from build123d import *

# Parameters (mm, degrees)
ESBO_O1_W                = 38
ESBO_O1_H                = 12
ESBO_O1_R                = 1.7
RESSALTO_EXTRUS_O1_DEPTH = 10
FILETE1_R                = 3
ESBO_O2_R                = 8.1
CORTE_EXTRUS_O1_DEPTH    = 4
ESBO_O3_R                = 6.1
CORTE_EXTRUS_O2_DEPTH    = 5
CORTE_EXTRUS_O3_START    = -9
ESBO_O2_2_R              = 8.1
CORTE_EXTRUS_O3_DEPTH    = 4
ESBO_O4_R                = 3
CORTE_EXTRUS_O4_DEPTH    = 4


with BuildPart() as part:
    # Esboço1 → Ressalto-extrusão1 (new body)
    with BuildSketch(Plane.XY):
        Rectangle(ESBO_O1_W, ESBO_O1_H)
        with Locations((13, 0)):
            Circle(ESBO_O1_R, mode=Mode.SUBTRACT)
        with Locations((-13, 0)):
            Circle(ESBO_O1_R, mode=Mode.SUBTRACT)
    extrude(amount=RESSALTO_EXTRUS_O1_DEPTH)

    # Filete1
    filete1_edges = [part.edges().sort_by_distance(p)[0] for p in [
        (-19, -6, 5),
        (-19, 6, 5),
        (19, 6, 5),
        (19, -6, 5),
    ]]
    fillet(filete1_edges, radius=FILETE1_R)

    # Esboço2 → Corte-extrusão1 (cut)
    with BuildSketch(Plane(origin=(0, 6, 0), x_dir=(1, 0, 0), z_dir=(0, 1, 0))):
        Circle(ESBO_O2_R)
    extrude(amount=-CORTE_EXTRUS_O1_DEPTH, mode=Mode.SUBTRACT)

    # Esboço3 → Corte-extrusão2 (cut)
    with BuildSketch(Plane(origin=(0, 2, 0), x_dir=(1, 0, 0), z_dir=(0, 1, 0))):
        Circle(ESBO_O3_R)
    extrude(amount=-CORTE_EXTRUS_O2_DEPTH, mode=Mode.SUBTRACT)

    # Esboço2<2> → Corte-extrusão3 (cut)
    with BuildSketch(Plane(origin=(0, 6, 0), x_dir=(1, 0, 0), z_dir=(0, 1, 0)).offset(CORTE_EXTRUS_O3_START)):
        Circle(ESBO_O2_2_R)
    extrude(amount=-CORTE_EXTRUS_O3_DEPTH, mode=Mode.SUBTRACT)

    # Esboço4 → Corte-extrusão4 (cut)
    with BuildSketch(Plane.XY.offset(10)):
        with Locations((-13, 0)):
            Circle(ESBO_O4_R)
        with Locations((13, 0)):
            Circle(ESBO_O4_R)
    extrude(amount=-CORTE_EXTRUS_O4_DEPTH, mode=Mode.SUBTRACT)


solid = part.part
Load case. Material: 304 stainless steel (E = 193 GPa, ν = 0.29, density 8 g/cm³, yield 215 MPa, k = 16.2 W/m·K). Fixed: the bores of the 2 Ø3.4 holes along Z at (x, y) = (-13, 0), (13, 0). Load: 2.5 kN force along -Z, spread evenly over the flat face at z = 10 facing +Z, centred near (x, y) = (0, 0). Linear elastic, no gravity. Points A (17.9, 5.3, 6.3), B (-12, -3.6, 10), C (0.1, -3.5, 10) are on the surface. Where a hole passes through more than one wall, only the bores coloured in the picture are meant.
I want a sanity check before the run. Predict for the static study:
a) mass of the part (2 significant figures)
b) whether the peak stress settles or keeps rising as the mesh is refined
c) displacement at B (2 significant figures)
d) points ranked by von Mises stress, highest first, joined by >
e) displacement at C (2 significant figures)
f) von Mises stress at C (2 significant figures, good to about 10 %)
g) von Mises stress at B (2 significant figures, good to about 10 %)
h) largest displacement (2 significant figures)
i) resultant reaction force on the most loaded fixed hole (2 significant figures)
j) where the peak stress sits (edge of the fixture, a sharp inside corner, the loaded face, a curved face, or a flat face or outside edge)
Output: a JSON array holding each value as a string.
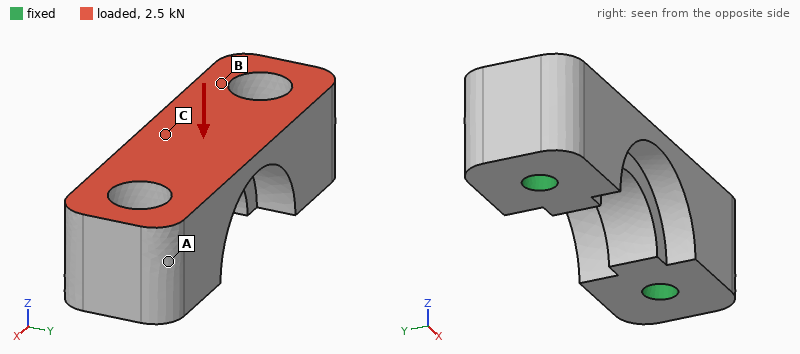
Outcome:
["25 g", "keeps rising", "0.90 µm", "C > B > A", "2.7 µm", "33 MPa", "13 MPa", "3.4 µm", "1.4 kN", "edge of the fixture"]
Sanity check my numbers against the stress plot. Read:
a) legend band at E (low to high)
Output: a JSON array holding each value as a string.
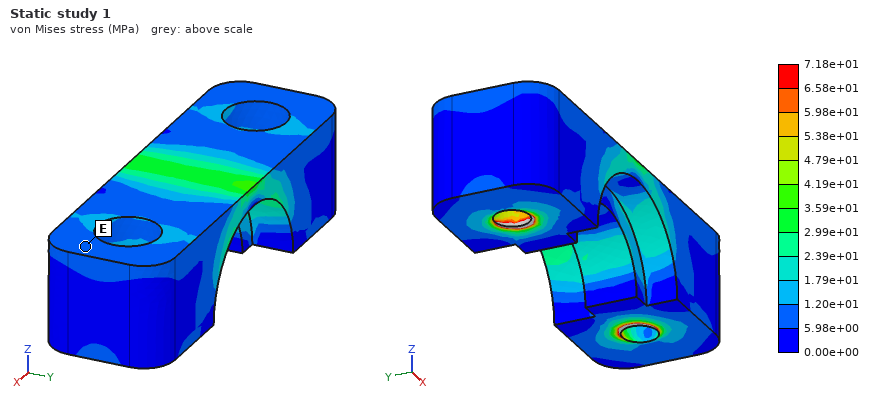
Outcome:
["5.98e+00 to 1.20e+01 MPa"]
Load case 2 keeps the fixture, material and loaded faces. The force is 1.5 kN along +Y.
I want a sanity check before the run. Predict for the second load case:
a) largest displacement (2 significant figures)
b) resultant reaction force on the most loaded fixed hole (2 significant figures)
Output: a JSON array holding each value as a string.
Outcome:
["5.7 µm", "750 N"]
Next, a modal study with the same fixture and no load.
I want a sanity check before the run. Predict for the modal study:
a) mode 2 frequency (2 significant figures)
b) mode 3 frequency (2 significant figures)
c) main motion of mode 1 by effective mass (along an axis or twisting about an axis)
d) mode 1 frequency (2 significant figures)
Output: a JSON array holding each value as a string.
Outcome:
["46 kHz", "47 kHz", "along Y", "32 kHz"]
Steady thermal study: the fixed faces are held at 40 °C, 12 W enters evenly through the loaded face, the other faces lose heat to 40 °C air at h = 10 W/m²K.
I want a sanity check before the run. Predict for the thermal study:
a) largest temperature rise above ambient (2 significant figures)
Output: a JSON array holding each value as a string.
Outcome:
["40 K"]
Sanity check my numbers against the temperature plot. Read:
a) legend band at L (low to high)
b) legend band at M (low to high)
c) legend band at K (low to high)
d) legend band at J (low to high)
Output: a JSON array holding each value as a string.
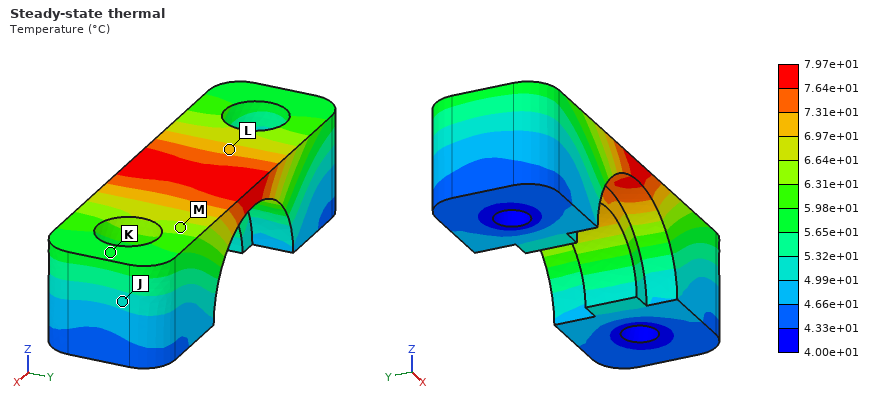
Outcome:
["6.97e+01 to 7.31e+01 °C", "6.31e+01 to 6.64e+01 °C", "5.65e+01 to 5.98e+01 °C", "4.99e+01 to 5.32e+01 °C"]
